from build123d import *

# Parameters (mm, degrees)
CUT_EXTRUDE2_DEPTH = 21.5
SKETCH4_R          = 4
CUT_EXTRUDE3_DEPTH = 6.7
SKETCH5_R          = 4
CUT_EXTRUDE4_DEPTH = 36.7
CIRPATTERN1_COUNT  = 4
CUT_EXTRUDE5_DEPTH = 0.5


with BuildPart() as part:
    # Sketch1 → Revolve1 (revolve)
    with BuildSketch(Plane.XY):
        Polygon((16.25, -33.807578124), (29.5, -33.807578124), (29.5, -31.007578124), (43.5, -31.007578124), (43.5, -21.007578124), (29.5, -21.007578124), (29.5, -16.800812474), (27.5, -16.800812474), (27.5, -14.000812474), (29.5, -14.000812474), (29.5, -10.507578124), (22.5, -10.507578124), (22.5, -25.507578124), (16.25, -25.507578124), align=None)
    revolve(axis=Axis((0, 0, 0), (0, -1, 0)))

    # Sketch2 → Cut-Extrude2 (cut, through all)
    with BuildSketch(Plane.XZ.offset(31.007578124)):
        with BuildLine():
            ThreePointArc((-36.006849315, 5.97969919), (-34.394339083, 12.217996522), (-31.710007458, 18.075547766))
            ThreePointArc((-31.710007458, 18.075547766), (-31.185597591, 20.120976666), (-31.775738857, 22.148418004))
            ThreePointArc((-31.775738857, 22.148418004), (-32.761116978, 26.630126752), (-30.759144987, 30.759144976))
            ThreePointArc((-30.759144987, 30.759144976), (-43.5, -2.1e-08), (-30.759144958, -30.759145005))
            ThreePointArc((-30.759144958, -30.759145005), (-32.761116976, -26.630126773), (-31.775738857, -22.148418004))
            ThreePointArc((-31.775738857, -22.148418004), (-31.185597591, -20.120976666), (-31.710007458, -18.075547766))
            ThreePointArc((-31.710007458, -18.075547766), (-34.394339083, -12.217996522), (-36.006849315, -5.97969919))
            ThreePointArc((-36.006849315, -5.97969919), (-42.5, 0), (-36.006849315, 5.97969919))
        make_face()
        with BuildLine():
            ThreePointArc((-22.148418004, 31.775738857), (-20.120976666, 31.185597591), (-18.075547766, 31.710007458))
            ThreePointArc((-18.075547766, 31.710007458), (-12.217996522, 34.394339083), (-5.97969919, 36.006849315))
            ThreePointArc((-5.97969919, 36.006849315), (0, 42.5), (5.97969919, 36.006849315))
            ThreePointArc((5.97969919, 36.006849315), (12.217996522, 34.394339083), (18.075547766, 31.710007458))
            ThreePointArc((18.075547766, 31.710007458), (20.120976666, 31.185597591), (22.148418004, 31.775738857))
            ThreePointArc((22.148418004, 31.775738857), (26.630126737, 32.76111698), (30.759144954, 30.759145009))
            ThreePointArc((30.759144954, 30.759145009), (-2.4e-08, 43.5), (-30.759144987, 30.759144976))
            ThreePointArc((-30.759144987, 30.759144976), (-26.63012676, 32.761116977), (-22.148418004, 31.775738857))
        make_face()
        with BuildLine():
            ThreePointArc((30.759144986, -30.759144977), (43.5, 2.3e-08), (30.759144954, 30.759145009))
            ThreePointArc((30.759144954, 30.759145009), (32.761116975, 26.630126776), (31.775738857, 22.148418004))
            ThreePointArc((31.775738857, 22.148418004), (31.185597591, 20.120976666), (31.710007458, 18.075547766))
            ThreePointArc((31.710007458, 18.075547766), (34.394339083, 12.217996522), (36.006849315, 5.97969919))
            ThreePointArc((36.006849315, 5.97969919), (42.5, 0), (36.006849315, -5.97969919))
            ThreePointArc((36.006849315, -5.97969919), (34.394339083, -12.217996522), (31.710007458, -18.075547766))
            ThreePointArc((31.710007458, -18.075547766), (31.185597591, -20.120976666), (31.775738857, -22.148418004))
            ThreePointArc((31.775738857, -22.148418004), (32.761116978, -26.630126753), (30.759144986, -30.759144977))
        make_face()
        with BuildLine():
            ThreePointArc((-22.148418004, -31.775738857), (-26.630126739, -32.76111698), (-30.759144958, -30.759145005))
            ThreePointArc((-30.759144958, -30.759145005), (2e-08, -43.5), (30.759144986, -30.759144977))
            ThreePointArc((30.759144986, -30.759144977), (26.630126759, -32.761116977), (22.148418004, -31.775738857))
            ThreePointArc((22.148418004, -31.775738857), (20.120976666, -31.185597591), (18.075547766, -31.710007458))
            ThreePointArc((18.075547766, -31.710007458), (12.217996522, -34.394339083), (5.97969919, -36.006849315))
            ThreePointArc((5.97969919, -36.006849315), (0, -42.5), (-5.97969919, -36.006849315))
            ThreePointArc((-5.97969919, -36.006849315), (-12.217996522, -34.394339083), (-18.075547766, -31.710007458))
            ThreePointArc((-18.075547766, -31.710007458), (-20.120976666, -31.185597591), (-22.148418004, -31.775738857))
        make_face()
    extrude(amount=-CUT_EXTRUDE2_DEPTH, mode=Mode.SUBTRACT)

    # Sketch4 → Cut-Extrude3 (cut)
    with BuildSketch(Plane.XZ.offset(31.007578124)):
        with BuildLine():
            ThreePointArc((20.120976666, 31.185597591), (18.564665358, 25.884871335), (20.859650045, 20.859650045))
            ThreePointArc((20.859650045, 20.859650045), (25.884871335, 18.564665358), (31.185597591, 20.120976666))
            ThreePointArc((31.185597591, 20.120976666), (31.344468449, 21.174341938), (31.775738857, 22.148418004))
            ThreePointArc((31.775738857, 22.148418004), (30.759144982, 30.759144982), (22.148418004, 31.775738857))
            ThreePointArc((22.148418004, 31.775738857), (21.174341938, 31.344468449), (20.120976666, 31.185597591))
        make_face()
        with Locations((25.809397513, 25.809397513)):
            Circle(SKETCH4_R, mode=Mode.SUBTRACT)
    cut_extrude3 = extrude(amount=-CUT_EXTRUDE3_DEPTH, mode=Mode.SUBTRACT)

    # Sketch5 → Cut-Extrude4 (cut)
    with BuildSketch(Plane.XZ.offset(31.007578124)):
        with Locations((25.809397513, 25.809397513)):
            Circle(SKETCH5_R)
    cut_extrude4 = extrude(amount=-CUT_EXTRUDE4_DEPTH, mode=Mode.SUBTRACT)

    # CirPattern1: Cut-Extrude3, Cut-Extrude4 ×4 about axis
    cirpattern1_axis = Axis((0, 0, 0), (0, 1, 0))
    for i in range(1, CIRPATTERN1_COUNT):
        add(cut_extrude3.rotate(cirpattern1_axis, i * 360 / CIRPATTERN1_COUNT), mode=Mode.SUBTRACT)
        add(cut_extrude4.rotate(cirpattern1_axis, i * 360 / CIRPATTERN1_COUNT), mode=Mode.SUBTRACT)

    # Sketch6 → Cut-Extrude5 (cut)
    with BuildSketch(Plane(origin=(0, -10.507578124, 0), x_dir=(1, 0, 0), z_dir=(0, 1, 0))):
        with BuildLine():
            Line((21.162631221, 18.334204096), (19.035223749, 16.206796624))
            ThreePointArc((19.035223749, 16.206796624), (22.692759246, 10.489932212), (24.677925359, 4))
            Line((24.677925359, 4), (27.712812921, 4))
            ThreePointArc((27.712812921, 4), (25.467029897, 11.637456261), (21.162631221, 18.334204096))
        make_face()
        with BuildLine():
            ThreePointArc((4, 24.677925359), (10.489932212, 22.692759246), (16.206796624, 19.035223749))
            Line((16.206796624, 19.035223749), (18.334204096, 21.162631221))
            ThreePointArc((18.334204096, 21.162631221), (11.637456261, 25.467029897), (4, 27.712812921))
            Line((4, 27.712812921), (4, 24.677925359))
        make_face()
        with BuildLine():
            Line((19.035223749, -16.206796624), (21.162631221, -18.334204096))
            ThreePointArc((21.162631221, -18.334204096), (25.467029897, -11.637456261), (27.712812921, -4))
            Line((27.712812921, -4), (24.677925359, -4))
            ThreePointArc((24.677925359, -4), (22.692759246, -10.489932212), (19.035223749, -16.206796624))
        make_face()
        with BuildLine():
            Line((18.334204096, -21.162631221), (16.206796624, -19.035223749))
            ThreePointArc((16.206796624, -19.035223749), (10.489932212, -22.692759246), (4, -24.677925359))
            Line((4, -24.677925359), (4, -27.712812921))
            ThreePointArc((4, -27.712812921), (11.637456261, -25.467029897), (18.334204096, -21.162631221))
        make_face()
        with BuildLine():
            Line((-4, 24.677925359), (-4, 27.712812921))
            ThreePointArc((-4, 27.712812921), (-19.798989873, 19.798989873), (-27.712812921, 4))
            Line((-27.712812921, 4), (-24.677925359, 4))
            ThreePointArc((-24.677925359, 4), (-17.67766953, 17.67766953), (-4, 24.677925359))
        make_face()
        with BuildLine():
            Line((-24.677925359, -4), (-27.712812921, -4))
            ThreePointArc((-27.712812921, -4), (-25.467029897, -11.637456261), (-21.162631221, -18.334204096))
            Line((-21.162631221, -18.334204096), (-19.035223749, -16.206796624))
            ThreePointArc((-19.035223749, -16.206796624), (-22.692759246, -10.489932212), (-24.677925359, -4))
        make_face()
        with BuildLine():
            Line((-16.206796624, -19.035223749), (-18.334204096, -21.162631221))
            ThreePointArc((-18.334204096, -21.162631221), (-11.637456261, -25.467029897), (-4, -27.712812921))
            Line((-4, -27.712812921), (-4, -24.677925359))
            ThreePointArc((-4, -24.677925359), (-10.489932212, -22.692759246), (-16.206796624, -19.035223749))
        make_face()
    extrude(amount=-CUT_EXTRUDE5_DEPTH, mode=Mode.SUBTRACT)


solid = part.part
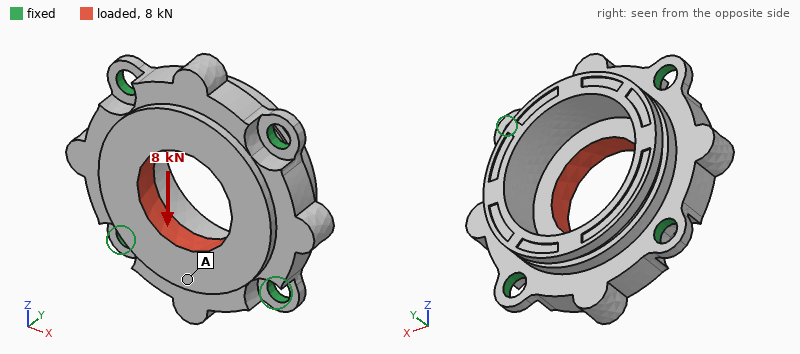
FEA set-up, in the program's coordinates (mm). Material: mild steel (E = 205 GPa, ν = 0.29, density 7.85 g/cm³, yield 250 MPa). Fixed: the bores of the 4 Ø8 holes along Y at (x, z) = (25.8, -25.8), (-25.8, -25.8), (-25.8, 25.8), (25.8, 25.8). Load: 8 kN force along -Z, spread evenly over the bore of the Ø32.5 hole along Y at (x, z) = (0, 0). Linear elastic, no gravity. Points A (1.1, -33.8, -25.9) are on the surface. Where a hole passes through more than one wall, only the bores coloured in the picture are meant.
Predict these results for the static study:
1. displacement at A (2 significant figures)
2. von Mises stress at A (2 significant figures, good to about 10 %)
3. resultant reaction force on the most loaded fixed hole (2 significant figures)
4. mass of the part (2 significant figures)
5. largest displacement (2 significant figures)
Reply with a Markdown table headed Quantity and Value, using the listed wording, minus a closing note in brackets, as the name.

| Quantity | Value |
|---|---|
| displacement at A | 4.2 µm |
| von Mises stress at A | 9.6 MPa |
| resultant reaction force on the most loaded fixed hole | 2.1 kN |
| mass of the part | 370 g |
| largest displacement | 4.6 µm |
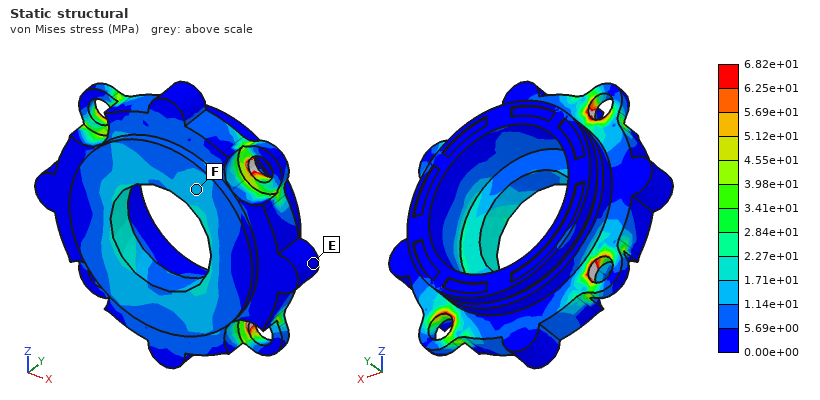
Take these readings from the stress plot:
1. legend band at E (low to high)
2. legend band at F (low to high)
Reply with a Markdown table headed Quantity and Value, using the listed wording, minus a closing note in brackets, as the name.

| Quantity | Value |
|---|---|
| legend band at E | 0.00e+00 to 5.69e+00 MPa |
| legend band at F | 1.14e+01 to 1.71e+01 MPa |
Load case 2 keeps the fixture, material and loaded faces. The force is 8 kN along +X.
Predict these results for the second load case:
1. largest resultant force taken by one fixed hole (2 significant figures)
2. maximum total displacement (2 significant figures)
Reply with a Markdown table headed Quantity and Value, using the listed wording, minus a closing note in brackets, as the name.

| Quantity | Value |
|---|---|
| largest resultant force taken by one fixed hole | 2.1 kN |
| maximum total displacement | 4.6 µm |
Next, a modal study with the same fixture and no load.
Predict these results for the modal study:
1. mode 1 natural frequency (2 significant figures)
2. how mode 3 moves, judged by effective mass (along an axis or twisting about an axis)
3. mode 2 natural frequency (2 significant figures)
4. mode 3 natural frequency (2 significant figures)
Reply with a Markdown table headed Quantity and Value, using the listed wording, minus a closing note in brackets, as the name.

| Quantity | Value |
|---|---|
| mode 1 natural frequency | 11 kHz |
| how mode 3 moves, judged by effective mass | twisting about X |
| mode 2 natural frequency | 11 kHz |
| mode 3 natural frequency | 12 kHz |
